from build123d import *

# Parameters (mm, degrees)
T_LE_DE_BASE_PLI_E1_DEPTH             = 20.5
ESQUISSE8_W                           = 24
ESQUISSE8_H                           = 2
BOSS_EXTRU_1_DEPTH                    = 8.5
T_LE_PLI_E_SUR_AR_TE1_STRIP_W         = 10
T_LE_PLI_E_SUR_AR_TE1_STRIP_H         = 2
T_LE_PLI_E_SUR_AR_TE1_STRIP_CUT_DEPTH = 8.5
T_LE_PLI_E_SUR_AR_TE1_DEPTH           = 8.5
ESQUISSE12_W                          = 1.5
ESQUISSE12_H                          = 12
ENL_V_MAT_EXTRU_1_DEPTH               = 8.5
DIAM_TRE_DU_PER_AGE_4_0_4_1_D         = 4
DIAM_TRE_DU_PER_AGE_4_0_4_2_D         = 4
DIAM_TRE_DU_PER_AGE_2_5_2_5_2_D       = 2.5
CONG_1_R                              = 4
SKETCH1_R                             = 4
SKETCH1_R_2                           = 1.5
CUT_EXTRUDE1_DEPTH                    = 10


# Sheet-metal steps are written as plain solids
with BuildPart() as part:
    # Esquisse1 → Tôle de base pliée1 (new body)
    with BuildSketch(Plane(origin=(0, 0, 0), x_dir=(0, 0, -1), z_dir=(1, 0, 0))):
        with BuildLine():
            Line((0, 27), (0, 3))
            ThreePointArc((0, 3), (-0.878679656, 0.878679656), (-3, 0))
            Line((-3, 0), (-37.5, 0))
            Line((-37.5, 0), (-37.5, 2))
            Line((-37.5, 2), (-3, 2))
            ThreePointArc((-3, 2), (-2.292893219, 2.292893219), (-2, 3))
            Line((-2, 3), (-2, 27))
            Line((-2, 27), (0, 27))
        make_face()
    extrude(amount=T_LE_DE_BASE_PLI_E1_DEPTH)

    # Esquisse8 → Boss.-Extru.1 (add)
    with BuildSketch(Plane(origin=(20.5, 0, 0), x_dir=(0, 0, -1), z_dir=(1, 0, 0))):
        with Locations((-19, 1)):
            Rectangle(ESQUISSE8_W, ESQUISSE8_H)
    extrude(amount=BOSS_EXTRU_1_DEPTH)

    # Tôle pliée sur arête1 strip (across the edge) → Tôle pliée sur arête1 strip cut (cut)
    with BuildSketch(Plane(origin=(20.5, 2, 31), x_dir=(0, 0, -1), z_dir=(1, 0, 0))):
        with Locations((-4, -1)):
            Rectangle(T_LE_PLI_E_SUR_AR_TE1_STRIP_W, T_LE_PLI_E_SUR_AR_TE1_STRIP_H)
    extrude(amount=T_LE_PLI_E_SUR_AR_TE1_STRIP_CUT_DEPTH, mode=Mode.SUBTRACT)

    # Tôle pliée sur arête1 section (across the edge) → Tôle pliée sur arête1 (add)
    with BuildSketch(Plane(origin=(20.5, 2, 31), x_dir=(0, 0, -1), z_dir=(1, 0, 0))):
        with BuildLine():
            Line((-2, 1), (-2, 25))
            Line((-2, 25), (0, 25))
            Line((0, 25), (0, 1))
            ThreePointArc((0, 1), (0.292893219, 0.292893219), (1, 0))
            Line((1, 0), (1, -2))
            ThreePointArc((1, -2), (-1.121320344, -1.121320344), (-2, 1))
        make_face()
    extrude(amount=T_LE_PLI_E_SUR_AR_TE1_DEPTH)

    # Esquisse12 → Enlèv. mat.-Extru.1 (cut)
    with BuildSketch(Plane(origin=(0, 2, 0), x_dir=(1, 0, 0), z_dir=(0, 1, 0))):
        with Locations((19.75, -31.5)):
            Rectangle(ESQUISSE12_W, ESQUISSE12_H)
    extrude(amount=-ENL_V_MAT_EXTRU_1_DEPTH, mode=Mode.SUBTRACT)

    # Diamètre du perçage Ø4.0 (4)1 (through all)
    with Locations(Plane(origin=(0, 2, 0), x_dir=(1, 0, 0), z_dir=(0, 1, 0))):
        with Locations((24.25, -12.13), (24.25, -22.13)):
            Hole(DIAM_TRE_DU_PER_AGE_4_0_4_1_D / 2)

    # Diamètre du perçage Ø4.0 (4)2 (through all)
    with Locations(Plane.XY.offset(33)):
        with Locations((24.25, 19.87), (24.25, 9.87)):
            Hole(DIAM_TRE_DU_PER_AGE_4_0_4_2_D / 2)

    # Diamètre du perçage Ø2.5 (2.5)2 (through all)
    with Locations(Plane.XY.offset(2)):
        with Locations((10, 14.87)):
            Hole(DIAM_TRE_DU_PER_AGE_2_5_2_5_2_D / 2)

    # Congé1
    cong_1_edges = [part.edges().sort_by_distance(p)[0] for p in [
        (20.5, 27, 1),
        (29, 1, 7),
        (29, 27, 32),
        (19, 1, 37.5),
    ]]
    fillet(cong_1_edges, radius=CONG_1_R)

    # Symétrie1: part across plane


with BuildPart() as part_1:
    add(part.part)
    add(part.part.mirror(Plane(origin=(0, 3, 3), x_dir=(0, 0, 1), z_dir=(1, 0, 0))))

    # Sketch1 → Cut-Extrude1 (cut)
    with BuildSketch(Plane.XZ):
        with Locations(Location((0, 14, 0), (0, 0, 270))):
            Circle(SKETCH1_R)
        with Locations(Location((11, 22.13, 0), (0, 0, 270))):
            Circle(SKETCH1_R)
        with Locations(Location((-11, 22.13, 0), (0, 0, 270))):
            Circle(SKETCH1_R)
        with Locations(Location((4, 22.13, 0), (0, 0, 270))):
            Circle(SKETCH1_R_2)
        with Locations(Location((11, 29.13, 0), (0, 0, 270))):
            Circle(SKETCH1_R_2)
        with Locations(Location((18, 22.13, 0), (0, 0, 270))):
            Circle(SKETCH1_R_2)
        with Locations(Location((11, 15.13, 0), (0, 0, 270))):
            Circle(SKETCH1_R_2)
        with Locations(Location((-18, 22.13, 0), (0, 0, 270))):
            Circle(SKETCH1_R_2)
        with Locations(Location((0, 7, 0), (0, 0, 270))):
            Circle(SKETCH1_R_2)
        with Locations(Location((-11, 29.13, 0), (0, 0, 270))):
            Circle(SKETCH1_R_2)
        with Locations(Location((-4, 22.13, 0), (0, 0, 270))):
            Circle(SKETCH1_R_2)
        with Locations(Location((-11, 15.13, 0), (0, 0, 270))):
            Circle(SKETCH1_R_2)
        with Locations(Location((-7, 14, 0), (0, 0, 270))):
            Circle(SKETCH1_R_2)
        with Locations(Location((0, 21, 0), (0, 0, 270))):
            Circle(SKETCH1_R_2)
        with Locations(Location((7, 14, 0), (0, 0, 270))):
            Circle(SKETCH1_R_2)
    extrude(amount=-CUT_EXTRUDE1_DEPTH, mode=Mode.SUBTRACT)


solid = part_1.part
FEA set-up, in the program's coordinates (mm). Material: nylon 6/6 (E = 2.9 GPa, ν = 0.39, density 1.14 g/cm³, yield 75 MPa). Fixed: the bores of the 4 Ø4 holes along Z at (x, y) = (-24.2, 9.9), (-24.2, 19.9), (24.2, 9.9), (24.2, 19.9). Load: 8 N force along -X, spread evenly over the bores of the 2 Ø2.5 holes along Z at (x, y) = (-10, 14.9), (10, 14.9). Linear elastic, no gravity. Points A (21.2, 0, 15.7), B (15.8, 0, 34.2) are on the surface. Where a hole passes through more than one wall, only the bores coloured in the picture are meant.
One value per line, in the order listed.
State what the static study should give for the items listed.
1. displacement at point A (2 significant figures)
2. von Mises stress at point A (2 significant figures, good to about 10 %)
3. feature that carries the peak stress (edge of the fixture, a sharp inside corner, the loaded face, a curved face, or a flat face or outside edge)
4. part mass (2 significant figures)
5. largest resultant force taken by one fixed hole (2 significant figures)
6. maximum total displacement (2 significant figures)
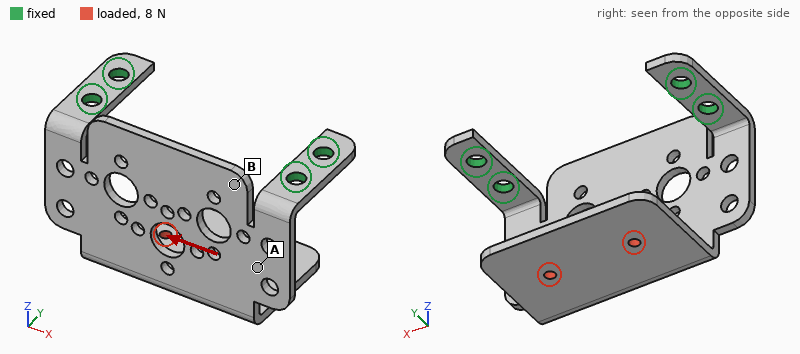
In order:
0.25 mm
2.4 MPa
a flat face or outside edge
6.8 g
7.0 N
0.77 mm
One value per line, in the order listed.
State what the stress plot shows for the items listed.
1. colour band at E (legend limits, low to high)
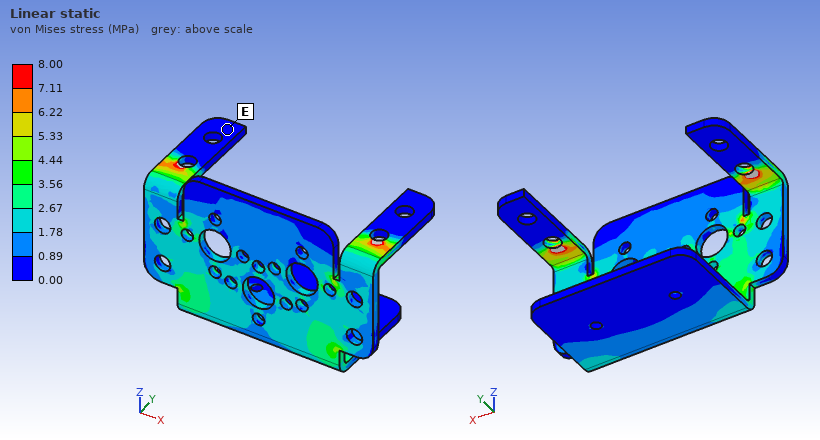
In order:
0.00 to 0.89 MPa
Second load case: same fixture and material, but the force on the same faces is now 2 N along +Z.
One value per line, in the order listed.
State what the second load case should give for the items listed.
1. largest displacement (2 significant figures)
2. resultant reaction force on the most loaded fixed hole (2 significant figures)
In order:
0.77 mm
1.0 N
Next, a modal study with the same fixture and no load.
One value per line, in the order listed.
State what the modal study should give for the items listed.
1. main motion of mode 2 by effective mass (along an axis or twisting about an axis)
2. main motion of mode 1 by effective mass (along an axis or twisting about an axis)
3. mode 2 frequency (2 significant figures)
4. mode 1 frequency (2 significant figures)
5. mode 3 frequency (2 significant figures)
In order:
along X
along Y
340 Hz
120 Hz
450 Hz
